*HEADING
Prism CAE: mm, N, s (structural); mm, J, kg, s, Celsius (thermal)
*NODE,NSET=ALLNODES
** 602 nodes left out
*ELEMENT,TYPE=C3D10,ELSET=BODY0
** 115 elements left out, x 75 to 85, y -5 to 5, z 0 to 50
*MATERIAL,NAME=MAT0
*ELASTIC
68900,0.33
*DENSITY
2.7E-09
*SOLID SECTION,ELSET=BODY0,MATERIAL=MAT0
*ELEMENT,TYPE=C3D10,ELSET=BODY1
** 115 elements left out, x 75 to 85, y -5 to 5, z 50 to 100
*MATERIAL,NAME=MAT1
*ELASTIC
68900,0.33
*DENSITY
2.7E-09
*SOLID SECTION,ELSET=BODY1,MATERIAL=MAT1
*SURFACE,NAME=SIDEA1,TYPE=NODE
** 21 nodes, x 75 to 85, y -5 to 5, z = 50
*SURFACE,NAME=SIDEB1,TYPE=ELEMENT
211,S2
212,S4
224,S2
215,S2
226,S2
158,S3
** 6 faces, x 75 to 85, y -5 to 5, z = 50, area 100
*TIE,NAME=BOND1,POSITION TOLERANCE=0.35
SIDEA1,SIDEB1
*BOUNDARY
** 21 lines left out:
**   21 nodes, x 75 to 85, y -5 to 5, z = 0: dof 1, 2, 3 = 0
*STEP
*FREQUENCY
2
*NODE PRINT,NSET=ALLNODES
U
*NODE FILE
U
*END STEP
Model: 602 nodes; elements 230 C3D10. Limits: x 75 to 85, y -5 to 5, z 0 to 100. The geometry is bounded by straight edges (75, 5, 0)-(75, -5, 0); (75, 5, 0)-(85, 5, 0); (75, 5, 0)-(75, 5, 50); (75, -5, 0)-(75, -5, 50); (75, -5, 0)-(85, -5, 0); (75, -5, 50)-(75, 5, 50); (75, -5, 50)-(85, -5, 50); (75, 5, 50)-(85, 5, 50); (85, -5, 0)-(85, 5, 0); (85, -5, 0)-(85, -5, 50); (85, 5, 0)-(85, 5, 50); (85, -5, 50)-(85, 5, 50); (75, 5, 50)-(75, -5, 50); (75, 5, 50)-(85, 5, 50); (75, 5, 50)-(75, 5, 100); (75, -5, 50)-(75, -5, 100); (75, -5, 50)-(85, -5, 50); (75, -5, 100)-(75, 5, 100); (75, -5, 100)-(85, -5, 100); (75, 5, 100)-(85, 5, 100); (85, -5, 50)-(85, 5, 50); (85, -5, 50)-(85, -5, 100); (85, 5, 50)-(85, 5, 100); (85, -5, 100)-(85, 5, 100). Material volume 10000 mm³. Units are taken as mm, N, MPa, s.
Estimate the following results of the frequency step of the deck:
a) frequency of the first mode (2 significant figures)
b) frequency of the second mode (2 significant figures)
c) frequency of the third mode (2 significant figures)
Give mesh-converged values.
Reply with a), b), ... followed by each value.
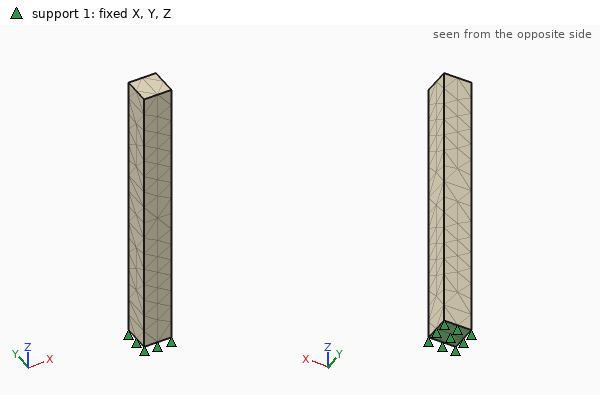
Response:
a) 820 Hz
b) 820 Hz
c) 4900 Hz
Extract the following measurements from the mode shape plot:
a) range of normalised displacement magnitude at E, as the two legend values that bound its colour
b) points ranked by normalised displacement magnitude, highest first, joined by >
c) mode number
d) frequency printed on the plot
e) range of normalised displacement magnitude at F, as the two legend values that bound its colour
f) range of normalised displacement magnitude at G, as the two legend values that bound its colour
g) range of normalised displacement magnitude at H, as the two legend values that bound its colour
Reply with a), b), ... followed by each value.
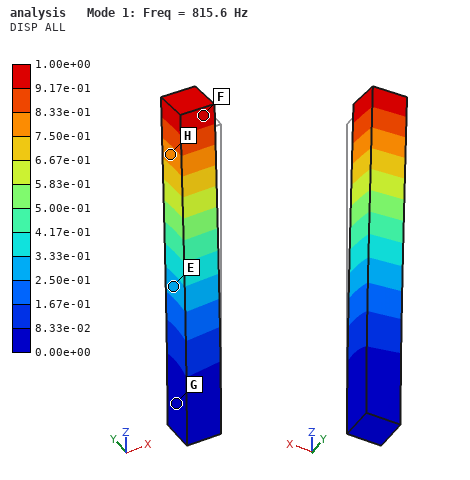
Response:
a) 2.50e-01 to 3.33e-01
b) F > H > E > G
c) 1
d) 815.6 Hz
e) 9.17e-01 to 1.00e+00
f) 0.00e+00 to 8.33e-02
g) 7.50e-01 to 8.33e-01
